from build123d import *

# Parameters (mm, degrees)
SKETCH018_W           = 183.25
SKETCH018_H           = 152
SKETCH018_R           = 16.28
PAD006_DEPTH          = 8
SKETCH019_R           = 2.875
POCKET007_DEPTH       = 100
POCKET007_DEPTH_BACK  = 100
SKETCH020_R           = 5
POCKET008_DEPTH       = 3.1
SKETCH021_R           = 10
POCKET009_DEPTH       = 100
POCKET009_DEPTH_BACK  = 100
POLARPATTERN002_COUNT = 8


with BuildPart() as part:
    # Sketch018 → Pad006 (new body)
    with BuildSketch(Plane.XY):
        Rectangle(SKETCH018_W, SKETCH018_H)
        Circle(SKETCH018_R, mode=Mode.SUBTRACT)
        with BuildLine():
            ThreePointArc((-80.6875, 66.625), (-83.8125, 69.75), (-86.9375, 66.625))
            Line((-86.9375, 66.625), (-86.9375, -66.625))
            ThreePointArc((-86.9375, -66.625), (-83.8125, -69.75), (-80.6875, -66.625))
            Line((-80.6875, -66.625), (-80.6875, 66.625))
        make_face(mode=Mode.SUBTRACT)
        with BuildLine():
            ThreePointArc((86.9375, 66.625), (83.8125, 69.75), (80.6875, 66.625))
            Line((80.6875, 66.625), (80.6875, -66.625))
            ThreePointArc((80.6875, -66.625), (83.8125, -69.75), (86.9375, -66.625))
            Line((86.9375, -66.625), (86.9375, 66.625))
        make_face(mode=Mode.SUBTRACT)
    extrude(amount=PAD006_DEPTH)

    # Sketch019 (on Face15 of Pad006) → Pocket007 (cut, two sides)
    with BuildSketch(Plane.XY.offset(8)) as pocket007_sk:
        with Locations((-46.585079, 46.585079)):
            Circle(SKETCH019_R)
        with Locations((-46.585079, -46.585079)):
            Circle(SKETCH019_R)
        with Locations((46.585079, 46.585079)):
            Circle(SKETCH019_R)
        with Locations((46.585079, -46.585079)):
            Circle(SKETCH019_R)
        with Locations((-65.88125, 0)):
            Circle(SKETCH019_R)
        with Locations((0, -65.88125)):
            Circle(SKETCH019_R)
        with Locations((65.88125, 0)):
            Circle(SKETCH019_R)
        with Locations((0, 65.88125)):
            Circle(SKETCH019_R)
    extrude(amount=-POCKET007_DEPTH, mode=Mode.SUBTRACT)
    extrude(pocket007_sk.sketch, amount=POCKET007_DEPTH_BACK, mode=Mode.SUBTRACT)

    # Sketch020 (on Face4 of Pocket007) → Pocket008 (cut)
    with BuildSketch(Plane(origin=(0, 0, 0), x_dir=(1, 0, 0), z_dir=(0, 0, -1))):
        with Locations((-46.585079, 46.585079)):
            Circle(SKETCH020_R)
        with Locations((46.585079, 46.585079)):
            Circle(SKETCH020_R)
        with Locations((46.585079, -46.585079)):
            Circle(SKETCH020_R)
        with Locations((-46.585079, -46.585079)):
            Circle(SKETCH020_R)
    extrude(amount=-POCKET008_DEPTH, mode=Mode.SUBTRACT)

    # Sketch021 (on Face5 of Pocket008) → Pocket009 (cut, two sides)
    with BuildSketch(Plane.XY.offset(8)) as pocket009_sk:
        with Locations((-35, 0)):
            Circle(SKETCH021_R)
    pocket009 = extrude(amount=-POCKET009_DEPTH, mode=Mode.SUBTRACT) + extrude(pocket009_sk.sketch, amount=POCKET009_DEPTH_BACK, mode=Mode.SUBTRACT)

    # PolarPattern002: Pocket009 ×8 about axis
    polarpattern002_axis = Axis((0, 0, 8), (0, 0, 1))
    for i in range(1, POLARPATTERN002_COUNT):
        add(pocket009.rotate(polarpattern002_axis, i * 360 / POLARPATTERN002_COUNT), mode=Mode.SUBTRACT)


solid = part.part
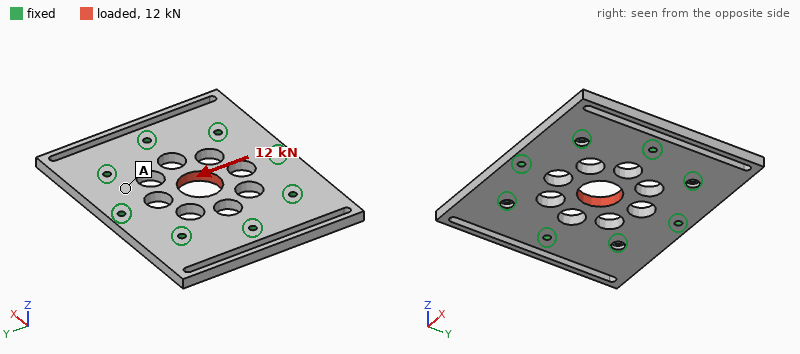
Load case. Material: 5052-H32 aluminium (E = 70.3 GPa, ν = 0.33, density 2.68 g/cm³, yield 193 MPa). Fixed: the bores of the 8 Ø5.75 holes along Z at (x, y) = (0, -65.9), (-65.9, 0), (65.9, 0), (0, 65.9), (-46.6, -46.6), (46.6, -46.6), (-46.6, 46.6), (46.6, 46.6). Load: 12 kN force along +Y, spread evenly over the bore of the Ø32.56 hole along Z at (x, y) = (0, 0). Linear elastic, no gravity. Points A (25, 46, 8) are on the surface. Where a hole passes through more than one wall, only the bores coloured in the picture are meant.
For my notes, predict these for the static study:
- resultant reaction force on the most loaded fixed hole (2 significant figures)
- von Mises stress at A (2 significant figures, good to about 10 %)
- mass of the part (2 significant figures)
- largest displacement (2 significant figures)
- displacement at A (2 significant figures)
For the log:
2.5 kN
10 MPa
480 g
19 µm
4.3 µm
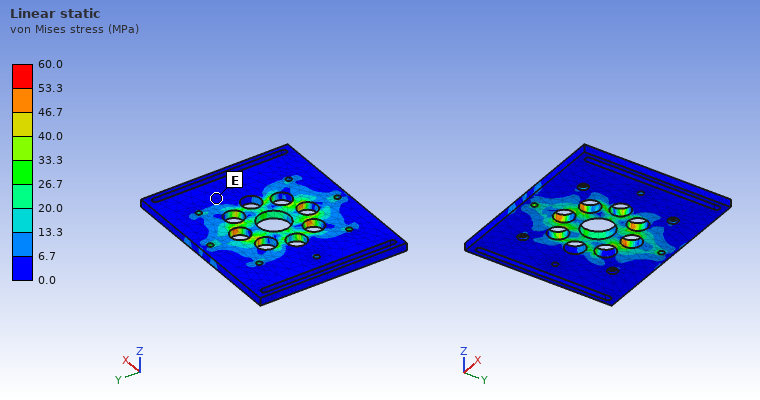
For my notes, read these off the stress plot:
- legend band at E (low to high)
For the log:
0.0 to 6.7 MPa
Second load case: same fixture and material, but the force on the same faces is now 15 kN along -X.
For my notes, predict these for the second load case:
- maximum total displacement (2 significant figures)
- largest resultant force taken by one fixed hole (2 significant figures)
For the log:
24 µm
3.2 kN
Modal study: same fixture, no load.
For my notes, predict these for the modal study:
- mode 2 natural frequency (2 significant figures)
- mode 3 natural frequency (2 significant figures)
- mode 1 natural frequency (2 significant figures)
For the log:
1200 Hz
1400 Hz
1200 Hz
